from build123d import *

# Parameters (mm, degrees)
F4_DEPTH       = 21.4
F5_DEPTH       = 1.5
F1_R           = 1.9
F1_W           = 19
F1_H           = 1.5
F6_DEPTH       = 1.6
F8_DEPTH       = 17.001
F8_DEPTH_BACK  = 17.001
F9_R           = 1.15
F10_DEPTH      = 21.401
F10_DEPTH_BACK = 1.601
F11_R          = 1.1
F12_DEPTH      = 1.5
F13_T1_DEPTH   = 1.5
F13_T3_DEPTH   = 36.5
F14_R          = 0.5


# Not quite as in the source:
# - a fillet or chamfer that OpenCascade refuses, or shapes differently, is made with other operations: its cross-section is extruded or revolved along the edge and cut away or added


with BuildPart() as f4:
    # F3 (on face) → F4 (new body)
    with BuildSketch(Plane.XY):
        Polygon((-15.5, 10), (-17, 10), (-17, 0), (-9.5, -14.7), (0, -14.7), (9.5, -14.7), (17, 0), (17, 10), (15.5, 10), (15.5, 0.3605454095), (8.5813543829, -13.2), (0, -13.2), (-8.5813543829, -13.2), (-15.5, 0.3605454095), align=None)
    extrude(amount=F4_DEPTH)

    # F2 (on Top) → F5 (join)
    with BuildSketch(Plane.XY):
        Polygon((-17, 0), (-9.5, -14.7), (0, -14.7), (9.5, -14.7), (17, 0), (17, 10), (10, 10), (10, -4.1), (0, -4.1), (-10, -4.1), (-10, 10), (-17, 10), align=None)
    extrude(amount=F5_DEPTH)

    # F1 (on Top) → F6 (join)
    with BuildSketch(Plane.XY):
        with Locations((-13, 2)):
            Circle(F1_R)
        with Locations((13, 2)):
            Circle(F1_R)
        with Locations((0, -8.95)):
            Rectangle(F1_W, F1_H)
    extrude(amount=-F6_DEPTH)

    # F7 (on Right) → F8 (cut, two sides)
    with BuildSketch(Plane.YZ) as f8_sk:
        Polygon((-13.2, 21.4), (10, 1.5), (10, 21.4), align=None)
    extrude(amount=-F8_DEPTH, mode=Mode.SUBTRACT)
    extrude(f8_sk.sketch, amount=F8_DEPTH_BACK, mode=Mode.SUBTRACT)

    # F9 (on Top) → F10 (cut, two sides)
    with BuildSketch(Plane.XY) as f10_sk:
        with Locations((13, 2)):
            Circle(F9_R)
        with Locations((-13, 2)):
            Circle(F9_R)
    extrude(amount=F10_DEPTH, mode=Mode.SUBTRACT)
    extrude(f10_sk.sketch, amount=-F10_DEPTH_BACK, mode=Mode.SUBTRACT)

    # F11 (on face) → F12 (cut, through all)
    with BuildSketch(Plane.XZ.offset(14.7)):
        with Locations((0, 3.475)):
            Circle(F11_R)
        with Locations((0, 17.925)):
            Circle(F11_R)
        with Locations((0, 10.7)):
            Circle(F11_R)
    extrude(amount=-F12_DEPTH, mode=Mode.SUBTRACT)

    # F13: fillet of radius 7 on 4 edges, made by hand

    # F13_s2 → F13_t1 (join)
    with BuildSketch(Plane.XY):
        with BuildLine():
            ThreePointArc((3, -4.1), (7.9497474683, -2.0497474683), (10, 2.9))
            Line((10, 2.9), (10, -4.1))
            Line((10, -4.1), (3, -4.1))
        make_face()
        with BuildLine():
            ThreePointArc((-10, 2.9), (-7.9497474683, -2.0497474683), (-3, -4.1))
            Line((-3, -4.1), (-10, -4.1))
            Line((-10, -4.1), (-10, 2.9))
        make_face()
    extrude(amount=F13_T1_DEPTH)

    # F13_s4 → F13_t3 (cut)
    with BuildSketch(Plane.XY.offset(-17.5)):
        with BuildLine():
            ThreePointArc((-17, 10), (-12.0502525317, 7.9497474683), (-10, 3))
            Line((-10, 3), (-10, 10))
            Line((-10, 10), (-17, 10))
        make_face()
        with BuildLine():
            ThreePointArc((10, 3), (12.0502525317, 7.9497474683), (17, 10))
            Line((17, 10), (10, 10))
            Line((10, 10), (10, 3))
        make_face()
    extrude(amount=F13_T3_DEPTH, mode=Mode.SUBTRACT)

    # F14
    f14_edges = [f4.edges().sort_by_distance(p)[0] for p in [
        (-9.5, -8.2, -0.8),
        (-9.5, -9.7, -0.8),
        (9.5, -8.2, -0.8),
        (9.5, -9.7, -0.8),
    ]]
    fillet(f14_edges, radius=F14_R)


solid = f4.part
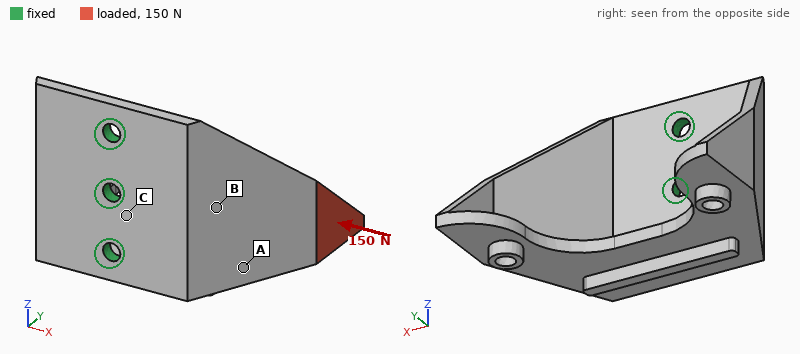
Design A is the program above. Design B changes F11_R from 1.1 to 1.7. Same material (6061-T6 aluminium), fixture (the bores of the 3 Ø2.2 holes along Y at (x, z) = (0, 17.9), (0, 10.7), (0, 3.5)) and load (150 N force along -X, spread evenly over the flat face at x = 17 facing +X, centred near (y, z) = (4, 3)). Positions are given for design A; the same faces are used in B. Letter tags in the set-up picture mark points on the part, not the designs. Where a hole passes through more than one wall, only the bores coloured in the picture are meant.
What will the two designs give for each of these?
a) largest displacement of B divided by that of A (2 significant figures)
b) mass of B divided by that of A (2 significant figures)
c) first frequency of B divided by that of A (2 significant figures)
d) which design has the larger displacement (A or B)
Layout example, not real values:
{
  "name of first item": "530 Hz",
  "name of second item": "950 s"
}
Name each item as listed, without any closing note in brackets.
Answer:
{
  "largest displacement of B divided by that of A": "0.69",
  "mass of B divided by that of A": "0.99",
  "first frequency of B divided by that of A": "1.3",
  "which design has the larger displacement": "A"
}
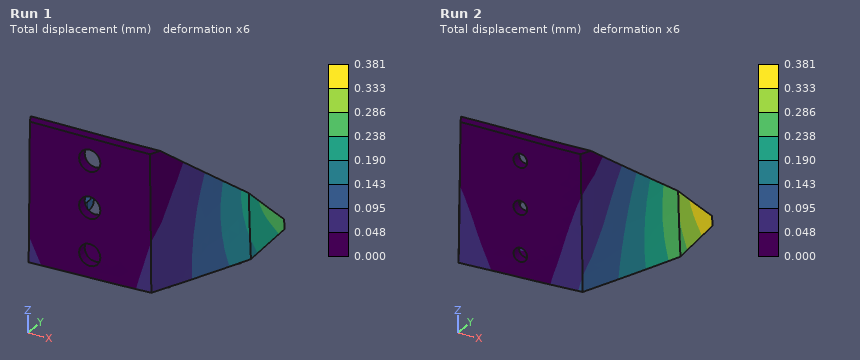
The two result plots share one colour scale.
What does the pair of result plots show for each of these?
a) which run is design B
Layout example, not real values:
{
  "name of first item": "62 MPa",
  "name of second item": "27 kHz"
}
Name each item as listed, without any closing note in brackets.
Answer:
{
  "which run is design B": "Run 1"
}
